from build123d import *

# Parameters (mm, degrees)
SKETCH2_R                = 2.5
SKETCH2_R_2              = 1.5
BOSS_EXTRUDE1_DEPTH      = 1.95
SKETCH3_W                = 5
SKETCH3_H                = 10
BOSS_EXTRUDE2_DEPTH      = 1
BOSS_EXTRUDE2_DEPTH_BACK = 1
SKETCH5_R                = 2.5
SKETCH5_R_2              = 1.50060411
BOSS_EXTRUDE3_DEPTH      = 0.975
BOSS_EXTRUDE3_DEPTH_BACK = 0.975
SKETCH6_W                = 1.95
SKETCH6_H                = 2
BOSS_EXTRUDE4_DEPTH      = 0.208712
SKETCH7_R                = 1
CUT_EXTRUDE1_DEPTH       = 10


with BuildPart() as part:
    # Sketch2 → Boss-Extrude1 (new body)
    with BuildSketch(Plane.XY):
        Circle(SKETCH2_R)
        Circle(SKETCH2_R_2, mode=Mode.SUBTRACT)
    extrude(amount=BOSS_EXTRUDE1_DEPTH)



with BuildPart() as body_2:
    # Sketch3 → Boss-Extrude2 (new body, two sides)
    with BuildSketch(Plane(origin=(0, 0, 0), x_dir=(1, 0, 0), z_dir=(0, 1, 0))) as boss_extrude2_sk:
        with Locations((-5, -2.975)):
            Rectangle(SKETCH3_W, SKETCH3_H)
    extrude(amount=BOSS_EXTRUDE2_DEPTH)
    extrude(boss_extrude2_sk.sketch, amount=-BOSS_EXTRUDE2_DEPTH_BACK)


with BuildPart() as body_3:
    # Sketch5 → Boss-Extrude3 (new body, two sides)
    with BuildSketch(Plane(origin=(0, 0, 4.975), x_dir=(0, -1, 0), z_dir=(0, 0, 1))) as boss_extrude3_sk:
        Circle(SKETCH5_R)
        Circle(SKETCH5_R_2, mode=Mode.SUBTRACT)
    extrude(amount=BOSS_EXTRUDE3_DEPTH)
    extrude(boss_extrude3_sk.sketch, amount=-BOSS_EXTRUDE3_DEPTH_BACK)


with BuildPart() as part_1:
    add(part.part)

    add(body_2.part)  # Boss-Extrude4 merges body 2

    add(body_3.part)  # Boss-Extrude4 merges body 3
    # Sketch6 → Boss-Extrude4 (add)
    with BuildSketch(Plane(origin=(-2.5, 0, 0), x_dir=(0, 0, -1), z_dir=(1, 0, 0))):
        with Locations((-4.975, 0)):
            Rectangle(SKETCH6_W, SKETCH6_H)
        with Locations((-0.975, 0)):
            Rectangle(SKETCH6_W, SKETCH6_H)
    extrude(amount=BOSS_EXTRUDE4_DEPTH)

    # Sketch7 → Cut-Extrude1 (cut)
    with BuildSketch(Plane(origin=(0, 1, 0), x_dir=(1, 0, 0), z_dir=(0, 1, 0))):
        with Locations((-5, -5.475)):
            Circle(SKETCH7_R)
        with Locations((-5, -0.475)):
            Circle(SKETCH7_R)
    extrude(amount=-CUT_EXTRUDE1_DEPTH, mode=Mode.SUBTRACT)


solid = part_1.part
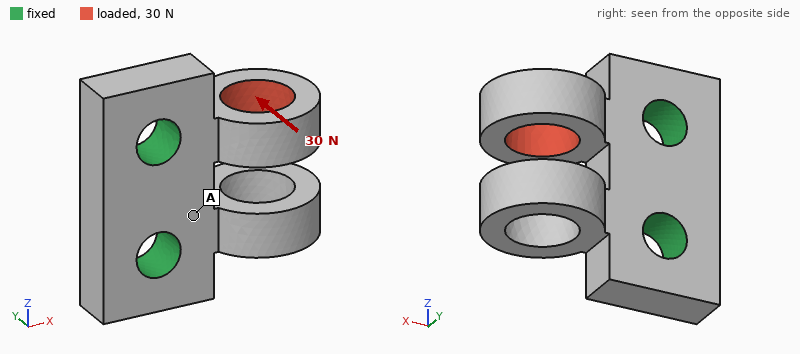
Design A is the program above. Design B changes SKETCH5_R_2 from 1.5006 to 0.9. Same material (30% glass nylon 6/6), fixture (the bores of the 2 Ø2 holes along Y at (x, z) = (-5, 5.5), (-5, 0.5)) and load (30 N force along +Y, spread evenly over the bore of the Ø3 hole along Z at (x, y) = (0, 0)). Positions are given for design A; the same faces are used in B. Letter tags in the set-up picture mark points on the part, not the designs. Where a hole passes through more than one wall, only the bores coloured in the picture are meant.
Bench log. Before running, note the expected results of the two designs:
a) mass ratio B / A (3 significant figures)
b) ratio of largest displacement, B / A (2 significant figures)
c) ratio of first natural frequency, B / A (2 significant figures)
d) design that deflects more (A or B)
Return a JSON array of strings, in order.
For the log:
["1.06", "0.66", "1.0", "A"]
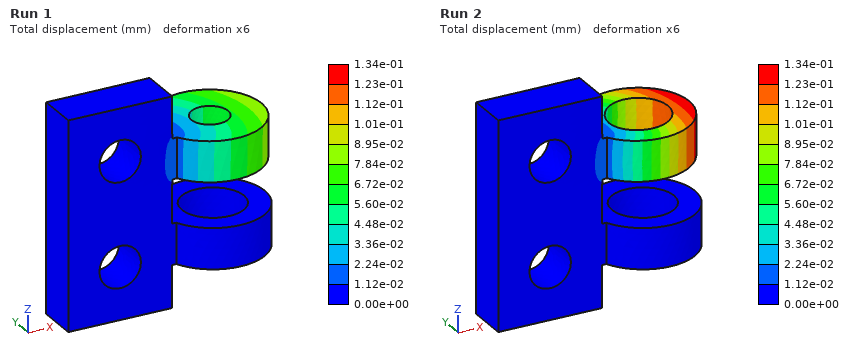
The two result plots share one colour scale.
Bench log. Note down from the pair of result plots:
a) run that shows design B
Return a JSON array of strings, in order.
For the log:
["Run 1"]
